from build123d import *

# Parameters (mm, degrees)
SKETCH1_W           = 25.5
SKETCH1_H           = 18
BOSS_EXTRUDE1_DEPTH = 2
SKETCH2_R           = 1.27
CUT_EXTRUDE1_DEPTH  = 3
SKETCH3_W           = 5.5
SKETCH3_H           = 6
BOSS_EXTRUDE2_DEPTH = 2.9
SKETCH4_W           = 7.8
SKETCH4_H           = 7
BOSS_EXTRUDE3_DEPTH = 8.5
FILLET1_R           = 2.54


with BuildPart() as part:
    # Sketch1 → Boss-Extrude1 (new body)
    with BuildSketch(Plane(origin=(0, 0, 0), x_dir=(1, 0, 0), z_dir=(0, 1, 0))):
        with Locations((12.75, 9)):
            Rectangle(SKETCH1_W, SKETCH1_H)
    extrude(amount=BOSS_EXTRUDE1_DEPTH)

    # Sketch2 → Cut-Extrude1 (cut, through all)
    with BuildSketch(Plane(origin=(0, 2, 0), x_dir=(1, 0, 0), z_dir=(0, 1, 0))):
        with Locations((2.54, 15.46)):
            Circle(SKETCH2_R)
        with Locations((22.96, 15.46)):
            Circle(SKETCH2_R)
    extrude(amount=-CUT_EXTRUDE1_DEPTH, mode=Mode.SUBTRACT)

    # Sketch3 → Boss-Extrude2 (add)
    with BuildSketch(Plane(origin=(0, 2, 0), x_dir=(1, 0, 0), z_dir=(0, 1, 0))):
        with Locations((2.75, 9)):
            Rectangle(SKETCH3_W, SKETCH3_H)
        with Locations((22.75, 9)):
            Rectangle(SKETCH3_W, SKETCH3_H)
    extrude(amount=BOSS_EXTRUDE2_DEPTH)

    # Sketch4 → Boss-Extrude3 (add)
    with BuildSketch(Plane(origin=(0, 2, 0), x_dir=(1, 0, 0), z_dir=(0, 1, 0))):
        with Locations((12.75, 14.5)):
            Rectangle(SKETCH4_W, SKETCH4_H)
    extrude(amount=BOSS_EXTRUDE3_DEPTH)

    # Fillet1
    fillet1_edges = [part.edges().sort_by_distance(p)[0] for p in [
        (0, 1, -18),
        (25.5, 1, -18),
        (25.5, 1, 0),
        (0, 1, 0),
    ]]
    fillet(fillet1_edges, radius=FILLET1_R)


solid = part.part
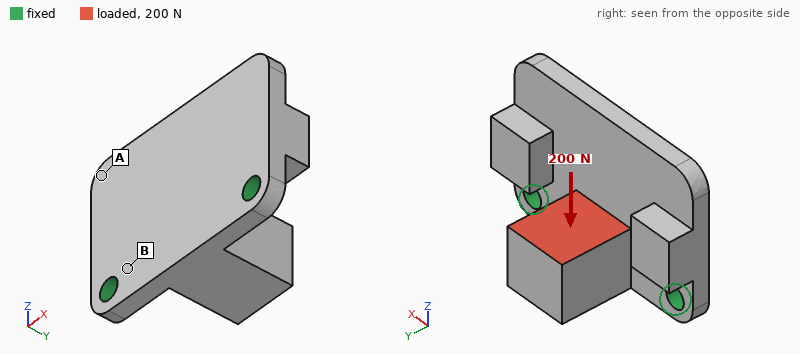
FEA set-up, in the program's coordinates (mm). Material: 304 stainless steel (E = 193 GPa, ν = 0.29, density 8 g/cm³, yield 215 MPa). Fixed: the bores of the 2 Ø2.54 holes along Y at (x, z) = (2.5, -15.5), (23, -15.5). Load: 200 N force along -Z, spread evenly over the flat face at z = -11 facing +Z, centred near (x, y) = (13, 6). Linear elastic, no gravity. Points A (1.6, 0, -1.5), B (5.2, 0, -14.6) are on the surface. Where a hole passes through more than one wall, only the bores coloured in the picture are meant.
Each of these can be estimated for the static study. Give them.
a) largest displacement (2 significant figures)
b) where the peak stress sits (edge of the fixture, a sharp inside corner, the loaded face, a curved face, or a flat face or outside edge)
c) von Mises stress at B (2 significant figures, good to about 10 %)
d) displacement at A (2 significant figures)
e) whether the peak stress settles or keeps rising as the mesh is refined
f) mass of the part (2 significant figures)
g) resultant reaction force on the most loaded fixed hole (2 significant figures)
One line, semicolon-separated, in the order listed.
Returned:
18 µm; edge of the fixture; 56 MPa; 13 µm; keeps rising; 12 g; 110 N
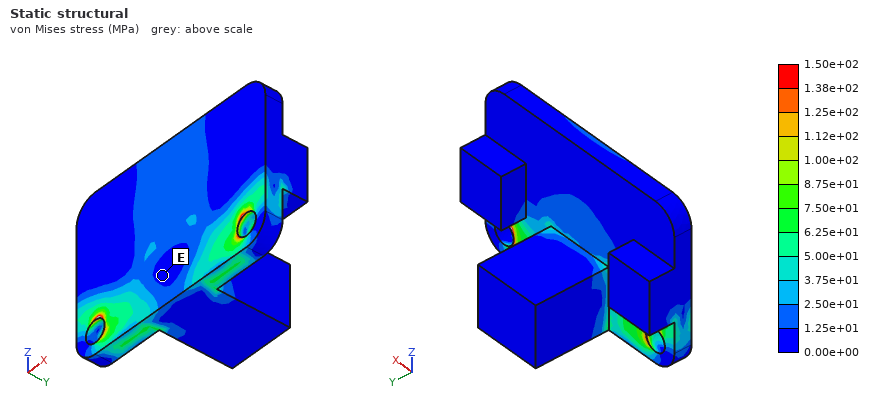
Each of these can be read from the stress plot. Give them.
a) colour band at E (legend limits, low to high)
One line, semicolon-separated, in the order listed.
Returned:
0.00e+00 to 1.25e+01 MPa
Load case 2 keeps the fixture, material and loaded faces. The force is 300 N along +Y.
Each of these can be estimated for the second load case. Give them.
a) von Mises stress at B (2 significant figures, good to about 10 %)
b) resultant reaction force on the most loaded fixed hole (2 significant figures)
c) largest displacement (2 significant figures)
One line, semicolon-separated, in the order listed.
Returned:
77 MPa; 150 N; 24 µm
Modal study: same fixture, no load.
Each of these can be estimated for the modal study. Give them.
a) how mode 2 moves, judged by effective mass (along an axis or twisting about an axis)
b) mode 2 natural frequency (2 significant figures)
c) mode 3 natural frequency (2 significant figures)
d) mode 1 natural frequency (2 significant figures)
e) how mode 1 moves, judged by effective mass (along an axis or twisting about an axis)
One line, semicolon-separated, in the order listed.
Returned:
twisting about Z; 13 kHz; 15 kHz; 5600 Hz; along Y
